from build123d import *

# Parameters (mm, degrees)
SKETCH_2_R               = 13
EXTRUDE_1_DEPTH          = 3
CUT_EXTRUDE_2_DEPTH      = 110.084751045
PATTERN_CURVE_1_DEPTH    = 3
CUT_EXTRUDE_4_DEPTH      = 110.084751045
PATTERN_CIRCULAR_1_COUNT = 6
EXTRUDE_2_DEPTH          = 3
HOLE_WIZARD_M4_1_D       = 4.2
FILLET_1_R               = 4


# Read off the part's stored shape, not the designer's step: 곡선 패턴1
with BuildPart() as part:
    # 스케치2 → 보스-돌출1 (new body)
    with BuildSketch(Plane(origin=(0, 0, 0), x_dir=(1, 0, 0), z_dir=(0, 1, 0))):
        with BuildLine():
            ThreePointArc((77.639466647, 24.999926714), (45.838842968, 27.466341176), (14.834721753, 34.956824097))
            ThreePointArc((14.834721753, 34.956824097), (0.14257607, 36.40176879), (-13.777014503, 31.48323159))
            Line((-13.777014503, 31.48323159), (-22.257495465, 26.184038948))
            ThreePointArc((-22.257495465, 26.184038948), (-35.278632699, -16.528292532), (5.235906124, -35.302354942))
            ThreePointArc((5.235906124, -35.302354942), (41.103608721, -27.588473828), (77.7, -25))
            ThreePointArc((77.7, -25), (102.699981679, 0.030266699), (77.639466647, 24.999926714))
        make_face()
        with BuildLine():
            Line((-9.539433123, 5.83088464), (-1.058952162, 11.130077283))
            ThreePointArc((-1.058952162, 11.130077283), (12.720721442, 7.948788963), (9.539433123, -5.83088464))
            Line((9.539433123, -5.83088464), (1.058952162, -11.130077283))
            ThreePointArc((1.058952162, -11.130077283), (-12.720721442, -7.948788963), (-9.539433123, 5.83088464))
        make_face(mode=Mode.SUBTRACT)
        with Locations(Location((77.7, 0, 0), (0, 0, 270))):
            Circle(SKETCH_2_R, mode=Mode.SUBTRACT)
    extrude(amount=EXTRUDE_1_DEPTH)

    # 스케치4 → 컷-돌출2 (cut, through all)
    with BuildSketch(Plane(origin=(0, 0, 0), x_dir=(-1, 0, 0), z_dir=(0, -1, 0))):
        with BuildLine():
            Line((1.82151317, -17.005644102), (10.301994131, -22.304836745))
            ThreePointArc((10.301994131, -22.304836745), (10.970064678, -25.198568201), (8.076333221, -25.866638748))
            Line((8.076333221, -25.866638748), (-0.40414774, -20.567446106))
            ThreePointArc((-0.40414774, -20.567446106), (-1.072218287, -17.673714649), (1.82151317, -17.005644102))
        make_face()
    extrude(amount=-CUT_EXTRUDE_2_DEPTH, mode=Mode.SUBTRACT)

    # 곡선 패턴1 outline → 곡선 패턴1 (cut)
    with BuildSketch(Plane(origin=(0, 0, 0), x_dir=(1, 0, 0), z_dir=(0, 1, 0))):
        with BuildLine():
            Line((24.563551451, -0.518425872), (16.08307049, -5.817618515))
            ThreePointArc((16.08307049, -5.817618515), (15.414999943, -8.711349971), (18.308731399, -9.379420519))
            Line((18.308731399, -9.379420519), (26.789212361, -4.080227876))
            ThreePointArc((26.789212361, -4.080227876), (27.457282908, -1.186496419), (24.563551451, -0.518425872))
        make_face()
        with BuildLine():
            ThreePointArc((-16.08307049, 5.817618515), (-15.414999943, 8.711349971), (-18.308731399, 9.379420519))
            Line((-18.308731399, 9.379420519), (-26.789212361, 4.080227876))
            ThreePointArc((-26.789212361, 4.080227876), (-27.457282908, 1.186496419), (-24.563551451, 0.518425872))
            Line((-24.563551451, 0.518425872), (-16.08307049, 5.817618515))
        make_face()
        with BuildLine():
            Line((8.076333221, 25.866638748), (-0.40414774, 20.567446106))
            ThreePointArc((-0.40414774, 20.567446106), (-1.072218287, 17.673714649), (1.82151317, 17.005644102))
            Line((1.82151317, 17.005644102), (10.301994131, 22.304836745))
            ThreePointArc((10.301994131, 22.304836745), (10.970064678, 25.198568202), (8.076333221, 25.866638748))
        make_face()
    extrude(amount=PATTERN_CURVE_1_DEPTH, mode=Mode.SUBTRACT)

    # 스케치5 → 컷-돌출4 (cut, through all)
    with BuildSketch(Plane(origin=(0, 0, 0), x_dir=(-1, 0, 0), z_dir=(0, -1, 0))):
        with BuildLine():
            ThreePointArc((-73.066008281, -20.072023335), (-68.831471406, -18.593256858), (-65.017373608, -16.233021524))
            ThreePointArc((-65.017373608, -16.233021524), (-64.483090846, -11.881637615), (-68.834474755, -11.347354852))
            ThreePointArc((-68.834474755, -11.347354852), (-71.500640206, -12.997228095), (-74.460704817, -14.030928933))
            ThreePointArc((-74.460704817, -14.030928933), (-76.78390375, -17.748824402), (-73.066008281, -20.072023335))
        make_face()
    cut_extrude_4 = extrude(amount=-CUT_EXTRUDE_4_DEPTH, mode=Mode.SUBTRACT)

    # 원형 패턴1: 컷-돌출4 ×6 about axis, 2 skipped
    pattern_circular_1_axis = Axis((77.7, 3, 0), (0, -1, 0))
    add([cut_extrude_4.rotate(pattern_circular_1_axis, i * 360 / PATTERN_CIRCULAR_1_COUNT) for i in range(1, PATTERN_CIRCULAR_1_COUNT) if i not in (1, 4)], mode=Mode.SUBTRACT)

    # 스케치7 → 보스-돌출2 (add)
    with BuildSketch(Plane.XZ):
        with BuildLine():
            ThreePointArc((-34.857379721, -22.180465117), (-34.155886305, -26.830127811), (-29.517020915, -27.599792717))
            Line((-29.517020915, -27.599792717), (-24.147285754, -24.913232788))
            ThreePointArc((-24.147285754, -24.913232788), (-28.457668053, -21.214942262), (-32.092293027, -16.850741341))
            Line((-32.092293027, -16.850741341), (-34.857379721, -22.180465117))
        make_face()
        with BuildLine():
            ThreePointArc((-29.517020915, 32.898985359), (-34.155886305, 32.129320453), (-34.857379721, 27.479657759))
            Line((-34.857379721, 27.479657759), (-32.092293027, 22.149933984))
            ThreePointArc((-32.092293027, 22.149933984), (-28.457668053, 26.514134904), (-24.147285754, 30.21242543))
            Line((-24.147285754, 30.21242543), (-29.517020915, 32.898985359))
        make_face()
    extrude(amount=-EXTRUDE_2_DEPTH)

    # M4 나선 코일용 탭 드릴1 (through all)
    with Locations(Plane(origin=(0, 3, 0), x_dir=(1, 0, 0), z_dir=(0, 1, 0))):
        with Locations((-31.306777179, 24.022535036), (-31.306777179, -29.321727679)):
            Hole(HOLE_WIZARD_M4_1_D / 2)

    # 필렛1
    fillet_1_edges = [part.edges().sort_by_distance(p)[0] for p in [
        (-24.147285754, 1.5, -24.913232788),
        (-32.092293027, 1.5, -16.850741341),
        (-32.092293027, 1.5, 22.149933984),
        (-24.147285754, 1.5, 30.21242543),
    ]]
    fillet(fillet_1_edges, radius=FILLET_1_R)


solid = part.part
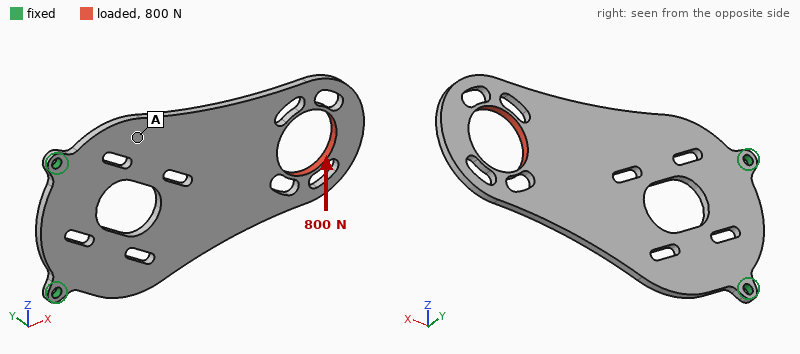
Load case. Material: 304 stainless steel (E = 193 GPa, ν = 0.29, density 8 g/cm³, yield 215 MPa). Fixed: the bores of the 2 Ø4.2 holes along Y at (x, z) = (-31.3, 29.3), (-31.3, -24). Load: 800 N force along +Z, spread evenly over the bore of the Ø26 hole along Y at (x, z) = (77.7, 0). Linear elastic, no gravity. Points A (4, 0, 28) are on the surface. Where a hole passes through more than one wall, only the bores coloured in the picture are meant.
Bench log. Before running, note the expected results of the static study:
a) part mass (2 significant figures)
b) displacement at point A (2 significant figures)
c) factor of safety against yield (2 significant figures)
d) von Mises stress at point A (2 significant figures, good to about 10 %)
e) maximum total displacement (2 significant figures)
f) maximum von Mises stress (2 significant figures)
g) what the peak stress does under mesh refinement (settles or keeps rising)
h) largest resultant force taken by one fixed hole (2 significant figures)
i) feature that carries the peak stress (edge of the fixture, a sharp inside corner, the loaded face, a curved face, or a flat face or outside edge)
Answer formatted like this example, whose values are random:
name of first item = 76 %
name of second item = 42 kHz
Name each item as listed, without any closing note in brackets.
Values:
part mass = 150 g
displacement at point A = 17 µm
factor of safety against yield = 1.2
von Mises stress at point A = 23 MPa
maximum total displacement = 83 µm
maximum von Mises stress = 180 MPa
what the peak stress does under mesh refinement = settles
largest resultant force taken by one fixed hole = 1.7 kN
feature that carries the peak stress = a curved face
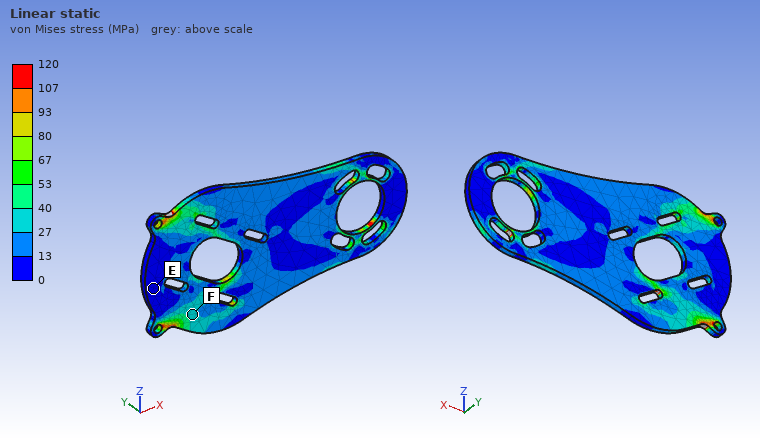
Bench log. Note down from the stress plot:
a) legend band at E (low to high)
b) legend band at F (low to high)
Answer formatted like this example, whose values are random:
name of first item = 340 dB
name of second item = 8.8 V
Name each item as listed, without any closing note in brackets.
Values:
legend band at E = 0 to 13 MPa
legend band at F = 27 to 40 MPa
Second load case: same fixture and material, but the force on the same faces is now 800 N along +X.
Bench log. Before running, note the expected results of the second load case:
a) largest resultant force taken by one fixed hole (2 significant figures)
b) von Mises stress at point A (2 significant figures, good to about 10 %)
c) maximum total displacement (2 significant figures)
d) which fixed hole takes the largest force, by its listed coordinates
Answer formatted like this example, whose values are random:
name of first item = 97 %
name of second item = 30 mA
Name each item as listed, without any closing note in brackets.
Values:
largest resultant force taken by one fixed hole = 450 N
von Mises stress at point A = 5.7 MPa
maximum total displacement = 10 µm
which fixed hole takes the largest force, by its listed coordinates = (-31.3, -24)
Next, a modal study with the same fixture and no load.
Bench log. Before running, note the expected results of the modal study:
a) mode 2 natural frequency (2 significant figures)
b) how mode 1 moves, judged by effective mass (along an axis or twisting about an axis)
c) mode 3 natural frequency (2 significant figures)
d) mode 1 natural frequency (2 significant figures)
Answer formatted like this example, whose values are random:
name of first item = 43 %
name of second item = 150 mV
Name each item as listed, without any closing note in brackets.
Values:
mode 2 natural frequency = 760 Hz
how mode 1 moves, judged by effective mass = along Y
mode 3 natural frequency = 810 Hz
mode 1 natural frequency = 150 Hz
